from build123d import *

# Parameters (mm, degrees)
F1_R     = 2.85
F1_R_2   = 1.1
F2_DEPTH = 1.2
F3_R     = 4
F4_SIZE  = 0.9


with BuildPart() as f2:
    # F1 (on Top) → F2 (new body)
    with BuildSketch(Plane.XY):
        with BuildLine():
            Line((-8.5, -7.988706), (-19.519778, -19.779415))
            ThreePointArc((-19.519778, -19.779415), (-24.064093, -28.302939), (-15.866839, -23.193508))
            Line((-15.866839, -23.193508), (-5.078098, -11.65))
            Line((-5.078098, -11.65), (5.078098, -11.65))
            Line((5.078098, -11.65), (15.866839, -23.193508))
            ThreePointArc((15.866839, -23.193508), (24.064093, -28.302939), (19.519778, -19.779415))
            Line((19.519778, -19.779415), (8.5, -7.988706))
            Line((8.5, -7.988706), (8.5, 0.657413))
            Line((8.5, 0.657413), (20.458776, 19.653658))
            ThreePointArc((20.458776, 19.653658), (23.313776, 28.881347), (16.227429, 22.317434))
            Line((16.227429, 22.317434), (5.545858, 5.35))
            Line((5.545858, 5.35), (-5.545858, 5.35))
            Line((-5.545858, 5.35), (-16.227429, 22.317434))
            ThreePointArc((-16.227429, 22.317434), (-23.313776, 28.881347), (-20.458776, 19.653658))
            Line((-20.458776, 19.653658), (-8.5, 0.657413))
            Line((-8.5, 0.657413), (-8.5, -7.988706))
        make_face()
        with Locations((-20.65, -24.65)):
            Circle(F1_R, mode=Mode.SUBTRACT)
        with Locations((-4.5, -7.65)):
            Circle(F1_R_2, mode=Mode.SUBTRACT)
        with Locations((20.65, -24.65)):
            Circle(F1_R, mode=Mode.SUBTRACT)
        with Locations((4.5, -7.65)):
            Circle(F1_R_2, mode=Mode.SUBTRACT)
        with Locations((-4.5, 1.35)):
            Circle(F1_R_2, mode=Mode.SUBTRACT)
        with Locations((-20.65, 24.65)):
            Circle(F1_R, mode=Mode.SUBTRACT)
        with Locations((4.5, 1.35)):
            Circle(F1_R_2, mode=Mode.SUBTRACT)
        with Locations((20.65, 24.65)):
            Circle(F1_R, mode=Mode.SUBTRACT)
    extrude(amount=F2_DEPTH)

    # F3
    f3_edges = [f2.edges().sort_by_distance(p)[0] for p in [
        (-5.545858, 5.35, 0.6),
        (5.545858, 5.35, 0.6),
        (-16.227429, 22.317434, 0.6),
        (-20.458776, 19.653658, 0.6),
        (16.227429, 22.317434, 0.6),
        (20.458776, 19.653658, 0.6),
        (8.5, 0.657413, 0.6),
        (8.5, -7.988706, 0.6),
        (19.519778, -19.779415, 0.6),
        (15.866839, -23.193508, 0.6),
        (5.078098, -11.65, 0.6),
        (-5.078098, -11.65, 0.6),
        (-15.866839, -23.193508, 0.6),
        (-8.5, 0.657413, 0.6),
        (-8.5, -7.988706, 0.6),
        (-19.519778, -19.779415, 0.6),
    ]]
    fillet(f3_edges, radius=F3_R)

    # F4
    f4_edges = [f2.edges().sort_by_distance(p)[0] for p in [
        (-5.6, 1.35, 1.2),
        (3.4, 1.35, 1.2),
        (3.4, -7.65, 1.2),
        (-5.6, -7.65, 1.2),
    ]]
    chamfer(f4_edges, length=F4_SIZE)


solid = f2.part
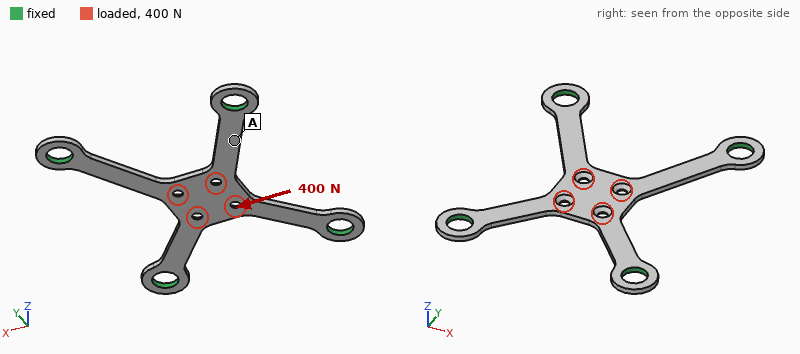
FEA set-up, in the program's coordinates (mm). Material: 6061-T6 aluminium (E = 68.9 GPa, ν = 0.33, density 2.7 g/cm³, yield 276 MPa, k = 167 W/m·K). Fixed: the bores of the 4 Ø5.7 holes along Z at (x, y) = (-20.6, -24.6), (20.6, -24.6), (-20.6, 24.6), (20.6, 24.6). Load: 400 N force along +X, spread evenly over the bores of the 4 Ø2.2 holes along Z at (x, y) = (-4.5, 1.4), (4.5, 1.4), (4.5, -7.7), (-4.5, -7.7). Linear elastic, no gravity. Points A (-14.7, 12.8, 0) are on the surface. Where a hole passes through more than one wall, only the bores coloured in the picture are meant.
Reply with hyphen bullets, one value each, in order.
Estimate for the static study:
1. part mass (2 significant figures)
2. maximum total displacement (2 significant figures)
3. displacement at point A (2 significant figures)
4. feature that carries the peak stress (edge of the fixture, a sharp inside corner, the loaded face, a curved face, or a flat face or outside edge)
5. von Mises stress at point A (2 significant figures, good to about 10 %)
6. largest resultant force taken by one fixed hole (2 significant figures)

- 2.6 g
- 42 µm
- 18 µm
- the loaded face
- 25 MPa
- 180 N
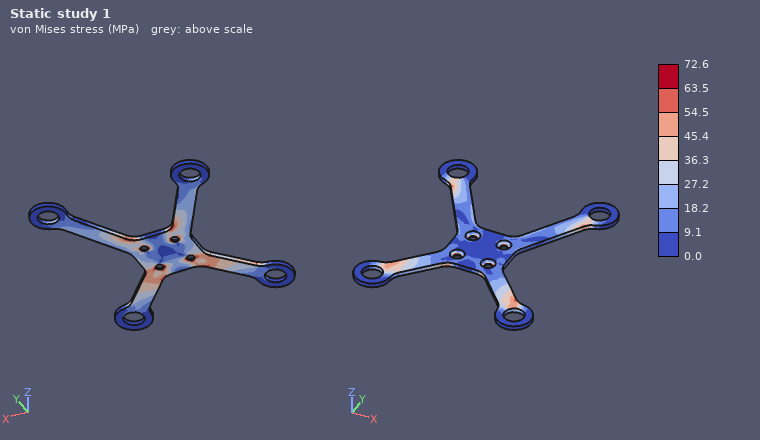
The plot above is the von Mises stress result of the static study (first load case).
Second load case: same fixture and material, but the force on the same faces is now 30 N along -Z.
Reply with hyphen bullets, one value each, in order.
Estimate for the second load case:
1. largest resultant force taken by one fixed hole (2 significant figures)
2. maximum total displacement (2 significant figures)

- 9.8 N
- 0.19 mm
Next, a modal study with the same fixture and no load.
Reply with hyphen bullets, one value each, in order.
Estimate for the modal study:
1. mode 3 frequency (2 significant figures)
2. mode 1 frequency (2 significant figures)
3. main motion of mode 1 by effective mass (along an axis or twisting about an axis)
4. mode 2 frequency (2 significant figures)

- 5300 Hz
- 2000 Hz
- along Z
- 4700 Hz
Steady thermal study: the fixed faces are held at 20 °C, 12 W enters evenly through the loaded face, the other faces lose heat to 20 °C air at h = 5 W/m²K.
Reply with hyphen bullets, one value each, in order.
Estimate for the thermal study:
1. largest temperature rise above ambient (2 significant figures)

- 70 K
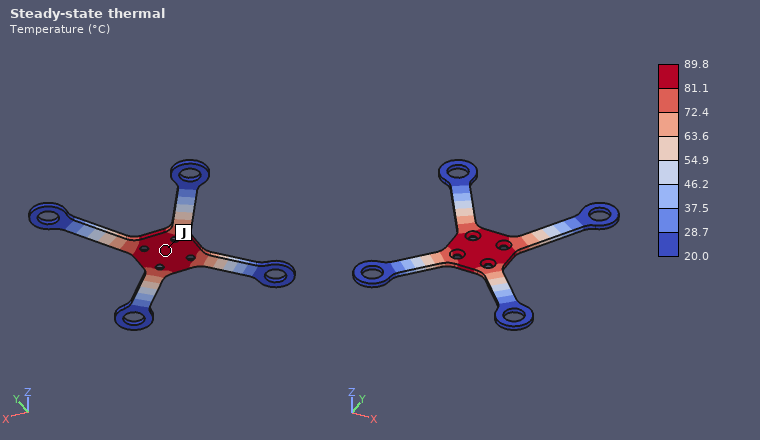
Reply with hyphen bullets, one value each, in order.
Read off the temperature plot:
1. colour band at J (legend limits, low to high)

- 81.1 to 89.8 °C
